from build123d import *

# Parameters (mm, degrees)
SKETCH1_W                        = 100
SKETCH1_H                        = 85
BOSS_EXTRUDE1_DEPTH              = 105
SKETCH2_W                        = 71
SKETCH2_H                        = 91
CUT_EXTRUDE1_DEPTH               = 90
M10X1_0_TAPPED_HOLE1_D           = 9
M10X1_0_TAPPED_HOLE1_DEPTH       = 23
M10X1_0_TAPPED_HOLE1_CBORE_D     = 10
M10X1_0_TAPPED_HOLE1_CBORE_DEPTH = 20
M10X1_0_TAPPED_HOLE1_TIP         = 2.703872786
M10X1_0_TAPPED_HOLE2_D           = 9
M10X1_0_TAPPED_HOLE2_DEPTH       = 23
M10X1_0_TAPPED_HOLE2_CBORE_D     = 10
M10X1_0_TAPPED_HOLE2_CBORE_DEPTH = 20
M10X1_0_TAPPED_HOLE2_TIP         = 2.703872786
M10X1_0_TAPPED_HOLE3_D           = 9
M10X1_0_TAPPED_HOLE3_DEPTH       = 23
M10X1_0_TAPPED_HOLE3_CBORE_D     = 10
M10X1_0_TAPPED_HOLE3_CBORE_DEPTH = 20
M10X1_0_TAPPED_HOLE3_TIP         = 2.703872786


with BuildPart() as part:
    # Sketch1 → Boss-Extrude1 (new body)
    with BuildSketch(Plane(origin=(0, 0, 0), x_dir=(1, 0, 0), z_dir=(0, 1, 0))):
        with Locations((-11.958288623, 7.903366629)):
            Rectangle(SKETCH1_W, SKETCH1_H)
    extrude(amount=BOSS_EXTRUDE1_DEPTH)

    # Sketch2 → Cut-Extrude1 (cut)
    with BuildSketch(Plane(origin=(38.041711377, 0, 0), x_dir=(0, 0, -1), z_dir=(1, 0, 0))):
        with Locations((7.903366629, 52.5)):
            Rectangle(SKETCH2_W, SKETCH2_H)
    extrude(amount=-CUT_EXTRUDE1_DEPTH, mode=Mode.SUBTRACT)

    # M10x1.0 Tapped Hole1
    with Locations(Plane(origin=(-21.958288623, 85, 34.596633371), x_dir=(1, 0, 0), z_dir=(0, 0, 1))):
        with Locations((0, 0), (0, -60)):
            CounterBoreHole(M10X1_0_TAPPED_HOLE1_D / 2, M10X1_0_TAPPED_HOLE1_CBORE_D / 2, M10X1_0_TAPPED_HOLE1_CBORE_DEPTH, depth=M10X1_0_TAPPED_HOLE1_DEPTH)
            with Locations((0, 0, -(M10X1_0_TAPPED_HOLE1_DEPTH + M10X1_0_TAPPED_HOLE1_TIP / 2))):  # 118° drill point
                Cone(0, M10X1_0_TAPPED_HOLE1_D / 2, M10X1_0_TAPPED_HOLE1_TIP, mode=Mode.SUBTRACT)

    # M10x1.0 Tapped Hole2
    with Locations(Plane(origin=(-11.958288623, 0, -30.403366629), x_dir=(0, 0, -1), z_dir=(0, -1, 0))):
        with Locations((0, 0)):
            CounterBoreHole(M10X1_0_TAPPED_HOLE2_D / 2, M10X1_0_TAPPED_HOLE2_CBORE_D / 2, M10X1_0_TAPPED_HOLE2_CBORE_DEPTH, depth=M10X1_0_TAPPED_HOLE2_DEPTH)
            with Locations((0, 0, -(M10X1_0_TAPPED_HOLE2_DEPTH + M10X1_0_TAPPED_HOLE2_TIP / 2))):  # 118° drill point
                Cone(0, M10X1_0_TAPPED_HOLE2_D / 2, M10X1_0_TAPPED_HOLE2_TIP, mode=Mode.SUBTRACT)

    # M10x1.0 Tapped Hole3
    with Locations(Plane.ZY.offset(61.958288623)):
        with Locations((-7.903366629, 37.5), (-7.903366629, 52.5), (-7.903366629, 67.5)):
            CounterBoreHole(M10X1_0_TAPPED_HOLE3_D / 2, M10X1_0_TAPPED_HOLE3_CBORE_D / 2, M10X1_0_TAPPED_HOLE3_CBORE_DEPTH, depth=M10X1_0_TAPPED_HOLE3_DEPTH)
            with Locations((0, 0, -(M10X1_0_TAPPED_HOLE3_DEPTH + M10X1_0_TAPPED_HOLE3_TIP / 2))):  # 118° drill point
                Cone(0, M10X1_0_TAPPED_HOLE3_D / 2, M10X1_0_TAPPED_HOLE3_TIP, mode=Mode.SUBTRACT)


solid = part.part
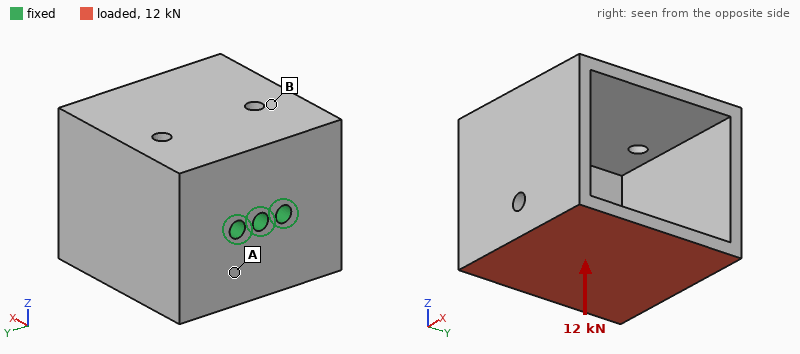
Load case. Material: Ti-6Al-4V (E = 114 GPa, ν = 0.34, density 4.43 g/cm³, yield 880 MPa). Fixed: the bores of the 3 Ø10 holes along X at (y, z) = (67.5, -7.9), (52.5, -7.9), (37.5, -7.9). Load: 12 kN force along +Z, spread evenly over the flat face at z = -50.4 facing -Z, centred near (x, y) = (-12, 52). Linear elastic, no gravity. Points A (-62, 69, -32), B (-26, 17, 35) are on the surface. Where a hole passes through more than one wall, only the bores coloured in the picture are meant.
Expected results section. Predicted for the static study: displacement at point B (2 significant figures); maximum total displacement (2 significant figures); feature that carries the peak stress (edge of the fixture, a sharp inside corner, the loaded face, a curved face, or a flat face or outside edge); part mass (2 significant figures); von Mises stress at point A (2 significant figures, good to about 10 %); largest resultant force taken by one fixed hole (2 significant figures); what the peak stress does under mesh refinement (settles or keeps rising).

0.22 mm
0.63 mm
edge of the fixture
1.4 kg
68 MPa
5.4 kN
keeps rising
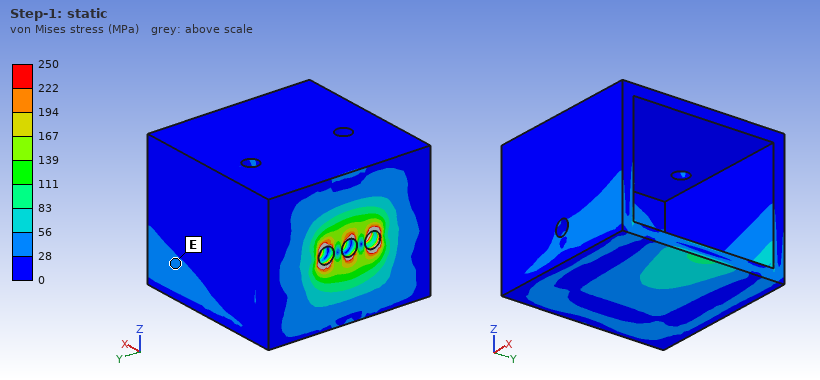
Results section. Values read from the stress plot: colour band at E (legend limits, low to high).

28 to 56 MPa
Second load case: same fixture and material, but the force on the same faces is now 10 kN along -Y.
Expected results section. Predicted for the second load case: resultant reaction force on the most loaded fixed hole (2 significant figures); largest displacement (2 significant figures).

14 kN
0.31 mm
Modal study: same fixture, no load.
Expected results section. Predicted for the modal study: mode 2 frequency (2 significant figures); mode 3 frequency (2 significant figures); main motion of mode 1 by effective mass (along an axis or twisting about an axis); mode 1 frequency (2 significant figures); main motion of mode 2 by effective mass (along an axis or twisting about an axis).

1100 Hz
1500 Hz
along Z
850 Hz
along Y
